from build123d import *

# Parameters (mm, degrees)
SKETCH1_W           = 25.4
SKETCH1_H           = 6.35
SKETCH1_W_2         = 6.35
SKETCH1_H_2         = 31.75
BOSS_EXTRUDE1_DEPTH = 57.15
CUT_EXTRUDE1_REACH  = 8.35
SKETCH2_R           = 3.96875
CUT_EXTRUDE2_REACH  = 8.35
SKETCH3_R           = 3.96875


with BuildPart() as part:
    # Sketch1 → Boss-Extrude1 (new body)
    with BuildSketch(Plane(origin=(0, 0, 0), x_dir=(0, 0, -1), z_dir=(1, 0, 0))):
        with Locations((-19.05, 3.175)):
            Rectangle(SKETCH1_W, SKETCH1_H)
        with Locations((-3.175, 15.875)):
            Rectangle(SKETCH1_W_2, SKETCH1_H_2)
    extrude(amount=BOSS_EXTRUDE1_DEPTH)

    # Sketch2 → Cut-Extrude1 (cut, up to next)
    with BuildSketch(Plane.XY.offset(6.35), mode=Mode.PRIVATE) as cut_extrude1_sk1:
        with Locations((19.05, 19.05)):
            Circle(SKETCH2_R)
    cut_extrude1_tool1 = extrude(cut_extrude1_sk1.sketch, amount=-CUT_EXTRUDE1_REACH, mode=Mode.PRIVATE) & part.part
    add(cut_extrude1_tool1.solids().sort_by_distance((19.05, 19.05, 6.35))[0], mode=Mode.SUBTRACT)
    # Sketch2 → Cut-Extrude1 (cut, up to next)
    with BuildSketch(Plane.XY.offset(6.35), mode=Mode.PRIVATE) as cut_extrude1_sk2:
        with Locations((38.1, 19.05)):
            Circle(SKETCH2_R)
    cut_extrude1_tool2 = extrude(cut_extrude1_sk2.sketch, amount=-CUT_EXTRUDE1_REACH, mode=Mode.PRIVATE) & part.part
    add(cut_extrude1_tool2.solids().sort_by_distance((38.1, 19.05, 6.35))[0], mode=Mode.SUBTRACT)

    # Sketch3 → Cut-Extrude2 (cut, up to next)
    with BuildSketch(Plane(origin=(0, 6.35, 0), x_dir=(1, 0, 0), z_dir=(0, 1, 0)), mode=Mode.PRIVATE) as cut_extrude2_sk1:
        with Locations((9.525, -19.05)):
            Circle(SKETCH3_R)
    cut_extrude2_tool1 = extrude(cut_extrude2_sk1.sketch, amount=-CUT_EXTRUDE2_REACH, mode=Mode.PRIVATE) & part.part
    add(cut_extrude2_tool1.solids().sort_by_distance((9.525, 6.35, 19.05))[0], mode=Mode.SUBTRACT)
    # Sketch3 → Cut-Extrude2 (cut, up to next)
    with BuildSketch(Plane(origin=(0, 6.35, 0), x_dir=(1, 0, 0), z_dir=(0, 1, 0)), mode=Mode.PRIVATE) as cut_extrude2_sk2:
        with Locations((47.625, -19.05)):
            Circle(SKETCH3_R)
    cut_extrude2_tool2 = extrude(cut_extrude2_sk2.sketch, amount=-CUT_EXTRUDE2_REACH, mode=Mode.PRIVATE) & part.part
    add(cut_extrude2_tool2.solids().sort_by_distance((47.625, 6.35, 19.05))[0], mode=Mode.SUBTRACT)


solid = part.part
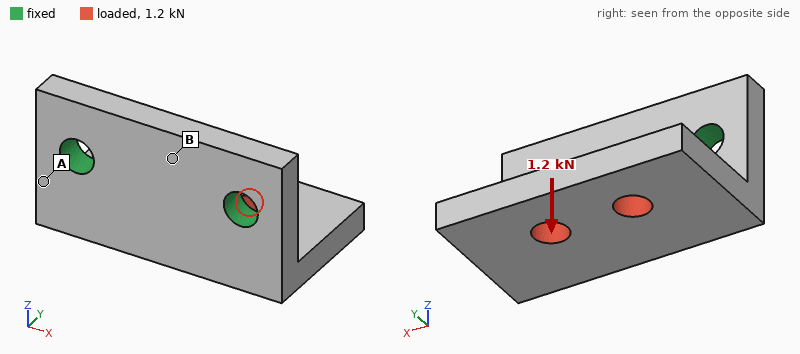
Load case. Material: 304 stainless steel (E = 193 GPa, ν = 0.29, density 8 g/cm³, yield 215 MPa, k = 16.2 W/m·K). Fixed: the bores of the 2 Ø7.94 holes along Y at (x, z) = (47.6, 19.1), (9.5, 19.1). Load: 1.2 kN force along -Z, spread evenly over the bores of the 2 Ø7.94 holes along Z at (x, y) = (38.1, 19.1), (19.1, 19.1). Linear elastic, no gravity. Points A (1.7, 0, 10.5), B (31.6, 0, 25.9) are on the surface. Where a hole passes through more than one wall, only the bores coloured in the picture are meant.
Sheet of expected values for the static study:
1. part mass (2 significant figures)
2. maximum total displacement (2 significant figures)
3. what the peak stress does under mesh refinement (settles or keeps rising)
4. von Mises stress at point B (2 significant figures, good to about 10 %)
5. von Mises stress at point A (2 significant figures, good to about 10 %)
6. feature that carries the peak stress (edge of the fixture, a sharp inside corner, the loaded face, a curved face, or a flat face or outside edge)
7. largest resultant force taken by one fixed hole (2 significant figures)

160 g
48 µm
keeps rising
8.7 MPa
48 MPa
edge of the fixture
620 N
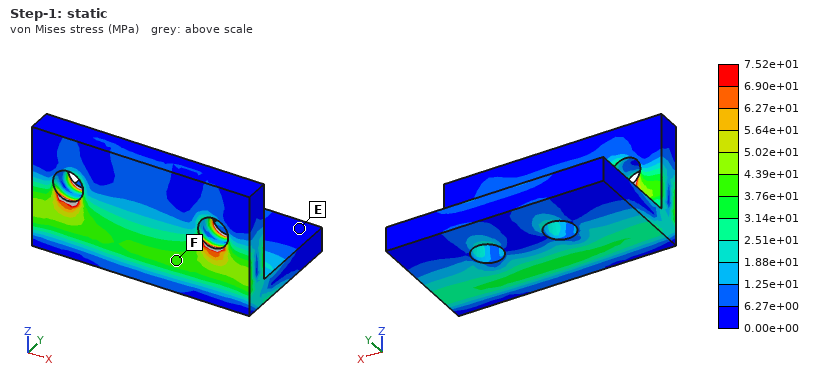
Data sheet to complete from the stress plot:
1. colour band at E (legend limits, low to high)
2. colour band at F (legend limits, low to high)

0.00e+00 to 6.27e+00 MPa
3.76e+01 to 4.39e+01 MPa
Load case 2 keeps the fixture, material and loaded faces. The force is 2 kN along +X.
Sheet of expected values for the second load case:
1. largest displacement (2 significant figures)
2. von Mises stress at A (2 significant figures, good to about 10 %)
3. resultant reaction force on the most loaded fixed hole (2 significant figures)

15 µm
20 MPa
1.4 kN
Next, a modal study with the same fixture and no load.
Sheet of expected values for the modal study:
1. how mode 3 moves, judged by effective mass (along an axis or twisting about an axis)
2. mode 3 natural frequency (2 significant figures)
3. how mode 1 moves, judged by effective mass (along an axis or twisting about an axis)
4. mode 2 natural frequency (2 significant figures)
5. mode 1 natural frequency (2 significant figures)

along X
9600 Hz
along Z
6200 Hz
3500 Hz
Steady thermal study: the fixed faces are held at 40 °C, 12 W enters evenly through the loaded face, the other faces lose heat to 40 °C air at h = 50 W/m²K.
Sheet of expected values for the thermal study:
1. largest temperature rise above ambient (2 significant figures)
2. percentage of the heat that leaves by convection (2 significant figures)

45 K
52 %
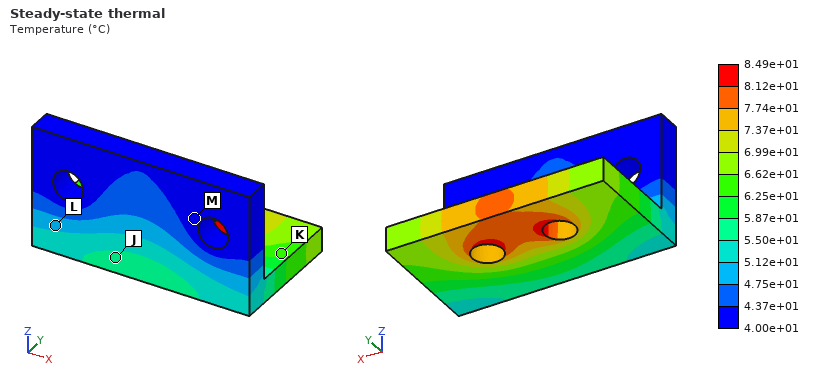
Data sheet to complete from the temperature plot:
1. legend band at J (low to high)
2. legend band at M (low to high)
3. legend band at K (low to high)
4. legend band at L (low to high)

5.50e+01 to 5.87e+01 °C
4.00e+01 to 4.37e+01 °C
6.25e+01 to 6.62e+01 °C
4.75e+01 to 5.12e+01 °C
